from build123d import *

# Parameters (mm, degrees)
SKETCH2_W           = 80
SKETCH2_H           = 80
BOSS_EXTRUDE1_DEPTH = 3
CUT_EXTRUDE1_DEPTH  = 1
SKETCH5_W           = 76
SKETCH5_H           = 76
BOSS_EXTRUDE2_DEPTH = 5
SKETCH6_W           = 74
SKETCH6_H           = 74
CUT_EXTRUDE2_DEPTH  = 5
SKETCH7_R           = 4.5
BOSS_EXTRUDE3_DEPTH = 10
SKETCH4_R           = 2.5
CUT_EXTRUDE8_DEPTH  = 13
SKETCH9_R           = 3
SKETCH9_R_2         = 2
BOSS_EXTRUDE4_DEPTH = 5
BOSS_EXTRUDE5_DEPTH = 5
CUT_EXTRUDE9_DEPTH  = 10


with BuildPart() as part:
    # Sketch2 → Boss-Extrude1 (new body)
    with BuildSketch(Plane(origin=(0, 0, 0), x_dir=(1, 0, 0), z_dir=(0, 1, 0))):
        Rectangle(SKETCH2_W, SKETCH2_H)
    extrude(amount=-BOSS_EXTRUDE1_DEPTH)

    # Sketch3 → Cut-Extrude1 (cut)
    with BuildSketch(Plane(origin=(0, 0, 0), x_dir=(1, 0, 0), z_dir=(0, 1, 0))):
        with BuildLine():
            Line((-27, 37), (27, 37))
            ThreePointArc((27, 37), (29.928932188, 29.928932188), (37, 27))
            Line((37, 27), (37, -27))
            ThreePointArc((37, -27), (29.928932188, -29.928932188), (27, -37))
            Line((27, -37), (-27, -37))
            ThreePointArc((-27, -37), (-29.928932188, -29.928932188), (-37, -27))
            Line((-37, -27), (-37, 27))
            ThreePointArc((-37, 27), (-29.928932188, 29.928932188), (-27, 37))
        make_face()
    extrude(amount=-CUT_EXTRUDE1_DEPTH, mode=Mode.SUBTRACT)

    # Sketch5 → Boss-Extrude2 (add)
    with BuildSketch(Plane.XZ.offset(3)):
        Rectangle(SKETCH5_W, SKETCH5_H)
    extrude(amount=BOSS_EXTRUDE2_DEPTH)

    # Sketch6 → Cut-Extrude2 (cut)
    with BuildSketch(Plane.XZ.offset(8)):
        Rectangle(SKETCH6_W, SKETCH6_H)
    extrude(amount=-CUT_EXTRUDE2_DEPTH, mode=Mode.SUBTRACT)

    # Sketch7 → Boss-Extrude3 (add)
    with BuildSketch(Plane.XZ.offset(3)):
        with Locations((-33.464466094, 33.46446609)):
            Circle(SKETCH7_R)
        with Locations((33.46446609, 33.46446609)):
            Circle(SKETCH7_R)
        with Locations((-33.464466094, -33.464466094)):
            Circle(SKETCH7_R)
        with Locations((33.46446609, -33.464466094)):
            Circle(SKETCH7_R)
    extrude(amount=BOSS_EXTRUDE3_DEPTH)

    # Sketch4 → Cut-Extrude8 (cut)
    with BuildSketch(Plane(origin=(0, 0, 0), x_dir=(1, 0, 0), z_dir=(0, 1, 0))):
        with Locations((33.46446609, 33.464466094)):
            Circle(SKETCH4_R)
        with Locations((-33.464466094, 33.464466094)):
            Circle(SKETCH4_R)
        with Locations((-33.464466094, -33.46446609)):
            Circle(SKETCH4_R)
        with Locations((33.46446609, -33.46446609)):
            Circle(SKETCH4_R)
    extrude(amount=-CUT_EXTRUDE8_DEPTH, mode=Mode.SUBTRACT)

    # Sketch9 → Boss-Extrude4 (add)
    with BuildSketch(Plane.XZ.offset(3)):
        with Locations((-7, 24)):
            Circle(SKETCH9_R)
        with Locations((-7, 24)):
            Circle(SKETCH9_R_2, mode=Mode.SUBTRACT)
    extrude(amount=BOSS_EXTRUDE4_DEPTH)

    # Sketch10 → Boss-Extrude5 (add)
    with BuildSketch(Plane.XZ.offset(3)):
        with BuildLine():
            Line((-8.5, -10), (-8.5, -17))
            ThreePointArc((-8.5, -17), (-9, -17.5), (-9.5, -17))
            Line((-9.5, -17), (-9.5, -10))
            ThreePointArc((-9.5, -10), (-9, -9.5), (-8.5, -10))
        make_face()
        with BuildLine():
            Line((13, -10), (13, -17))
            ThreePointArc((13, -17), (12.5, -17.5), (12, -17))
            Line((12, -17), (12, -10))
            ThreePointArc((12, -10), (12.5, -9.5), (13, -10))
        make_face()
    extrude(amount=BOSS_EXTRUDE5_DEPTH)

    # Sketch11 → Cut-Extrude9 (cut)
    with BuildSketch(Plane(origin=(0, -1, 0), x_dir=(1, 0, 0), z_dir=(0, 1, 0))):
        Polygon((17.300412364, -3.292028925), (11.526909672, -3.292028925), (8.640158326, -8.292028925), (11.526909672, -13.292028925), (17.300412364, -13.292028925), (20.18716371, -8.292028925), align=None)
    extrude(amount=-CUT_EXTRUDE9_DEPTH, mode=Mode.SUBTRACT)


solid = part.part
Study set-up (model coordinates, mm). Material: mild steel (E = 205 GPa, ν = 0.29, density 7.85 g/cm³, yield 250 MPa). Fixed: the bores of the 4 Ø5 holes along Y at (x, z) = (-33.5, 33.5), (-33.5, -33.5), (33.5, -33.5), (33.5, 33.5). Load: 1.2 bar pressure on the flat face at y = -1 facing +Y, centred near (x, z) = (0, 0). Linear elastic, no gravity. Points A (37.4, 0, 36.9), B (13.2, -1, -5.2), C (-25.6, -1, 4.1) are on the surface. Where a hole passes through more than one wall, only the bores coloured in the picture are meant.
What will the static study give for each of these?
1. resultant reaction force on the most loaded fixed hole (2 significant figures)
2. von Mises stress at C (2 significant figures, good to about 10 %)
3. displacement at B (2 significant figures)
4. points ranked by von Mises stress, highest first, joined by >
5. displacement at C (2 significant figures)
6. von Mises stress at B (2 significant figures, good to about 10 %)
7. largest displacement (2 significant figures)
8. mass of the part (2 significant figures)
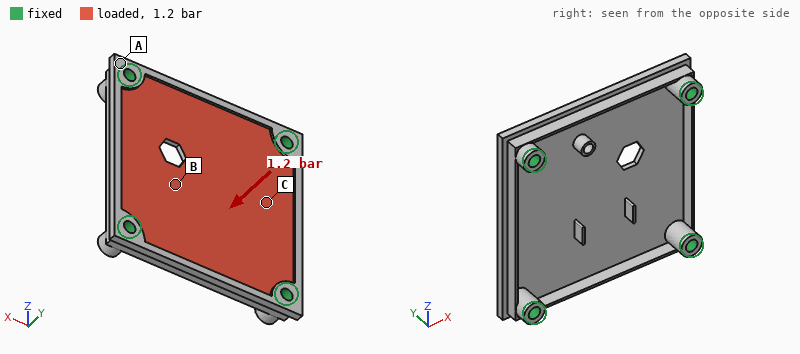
150 N
18 MPa
55 µm
B > C > A
32 µm
27 MPa
66 µm
130 g
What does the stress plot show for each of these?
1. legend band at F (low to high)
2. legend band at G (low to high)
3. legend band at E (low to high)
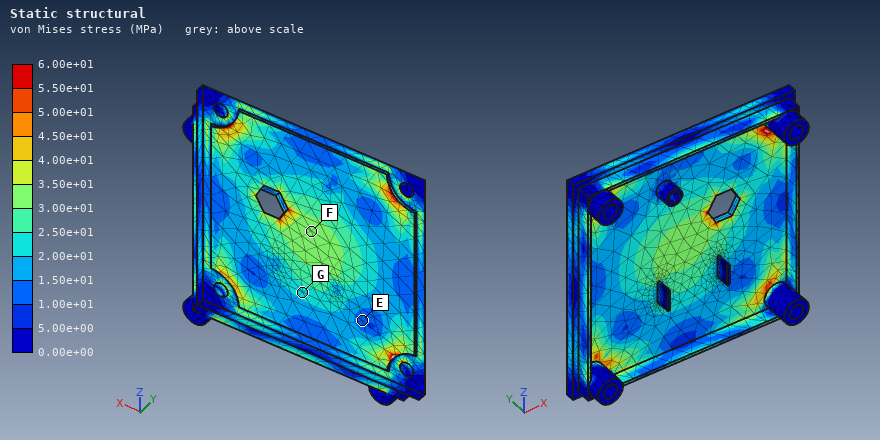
3.00e+01 to 3.50e+01 MPa
2.00e+01 to 2.50e+01 MPa
1.00e+01 to 1.50e+01 MPa
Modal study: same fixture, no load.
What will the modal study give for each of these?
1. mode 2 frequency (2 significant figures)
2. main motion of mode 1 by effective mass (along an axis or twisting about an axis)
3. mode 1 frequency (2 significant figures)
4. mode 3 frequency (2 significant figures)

4500 Hz
along Y
2100 Hz
4500 Hz
